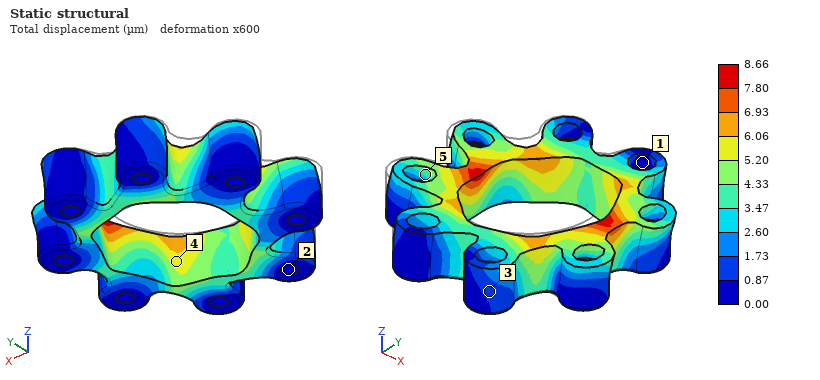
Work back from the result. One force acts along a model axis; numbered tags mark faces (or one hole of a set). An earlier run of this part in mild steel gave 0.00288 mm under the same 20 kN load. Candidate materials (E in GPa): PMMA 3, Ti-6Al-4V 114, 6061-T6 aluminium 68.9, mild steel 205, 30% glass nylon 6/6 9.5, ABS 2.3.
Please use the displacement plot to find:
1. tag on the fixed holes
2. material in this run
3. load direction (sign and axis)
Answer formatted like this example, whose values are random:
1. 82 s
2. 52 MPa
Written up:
1. 2
2. 6061-T6 aluminium
3. +X
